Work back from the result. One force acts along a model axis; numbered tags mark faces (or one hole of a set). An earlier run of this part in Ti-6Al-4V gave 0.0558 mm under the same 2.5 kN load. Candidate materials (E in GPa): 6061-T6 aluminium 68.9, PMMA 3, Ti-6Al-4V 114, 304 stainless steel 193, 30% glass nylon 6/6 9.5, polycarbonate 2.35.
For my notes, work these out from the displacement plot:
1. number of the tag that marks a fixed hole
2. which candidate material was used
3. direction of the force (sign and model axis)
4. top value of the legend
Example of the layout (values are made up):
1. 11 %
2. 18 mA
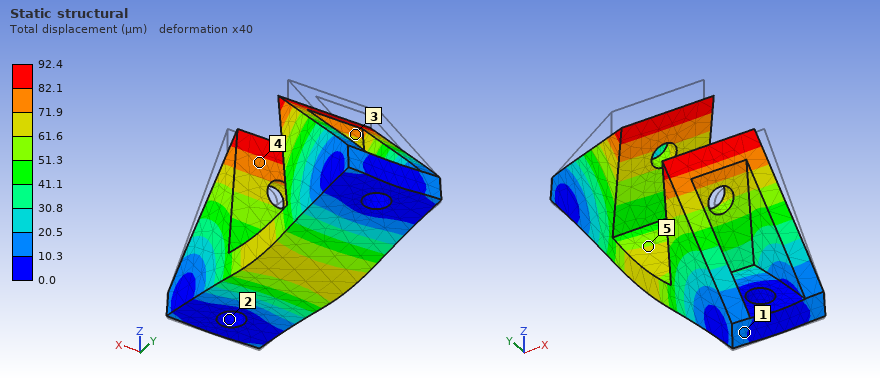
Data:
1. 2
2. 6061-T6 aluminium
3. -Z
4. 92.4 µm
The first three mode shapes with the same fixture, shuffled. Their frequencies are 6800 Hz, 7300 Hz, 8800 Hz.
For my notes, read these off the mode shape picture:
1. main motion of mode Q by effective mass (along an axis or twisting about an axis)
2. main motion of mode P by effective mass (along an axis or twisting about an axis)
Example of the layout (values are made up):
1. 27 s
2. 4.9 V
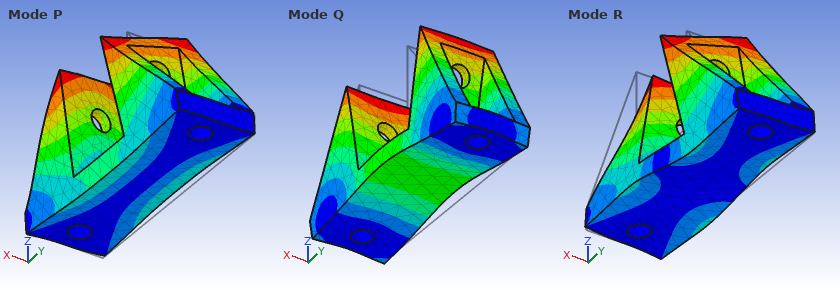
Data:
1. along Z
2. along X
